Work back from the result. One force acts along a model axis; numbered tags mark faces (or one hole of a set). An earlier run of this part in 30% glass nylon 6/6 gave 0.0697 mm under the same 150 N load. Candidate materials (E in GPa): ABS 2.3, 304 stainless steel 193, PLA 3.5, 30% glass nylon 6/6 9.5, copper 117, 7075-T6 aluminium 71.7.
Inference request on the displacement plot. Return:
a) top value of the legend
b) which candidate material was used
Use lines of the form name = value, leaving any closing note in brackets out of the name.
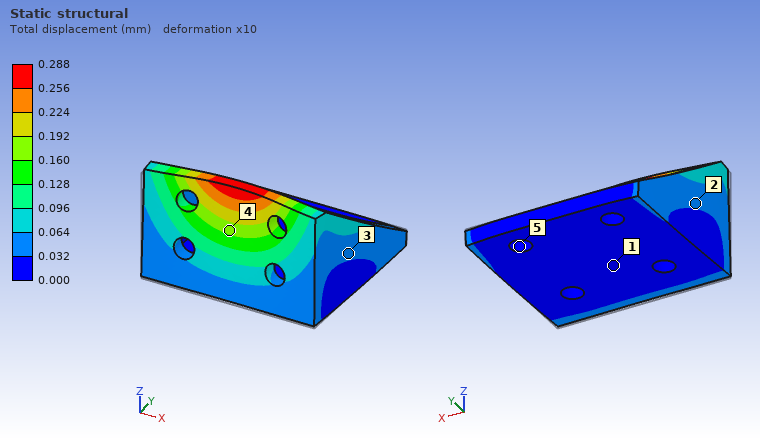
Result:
top value of the legend = 0.288 mm
which candidate material was used = ABS
